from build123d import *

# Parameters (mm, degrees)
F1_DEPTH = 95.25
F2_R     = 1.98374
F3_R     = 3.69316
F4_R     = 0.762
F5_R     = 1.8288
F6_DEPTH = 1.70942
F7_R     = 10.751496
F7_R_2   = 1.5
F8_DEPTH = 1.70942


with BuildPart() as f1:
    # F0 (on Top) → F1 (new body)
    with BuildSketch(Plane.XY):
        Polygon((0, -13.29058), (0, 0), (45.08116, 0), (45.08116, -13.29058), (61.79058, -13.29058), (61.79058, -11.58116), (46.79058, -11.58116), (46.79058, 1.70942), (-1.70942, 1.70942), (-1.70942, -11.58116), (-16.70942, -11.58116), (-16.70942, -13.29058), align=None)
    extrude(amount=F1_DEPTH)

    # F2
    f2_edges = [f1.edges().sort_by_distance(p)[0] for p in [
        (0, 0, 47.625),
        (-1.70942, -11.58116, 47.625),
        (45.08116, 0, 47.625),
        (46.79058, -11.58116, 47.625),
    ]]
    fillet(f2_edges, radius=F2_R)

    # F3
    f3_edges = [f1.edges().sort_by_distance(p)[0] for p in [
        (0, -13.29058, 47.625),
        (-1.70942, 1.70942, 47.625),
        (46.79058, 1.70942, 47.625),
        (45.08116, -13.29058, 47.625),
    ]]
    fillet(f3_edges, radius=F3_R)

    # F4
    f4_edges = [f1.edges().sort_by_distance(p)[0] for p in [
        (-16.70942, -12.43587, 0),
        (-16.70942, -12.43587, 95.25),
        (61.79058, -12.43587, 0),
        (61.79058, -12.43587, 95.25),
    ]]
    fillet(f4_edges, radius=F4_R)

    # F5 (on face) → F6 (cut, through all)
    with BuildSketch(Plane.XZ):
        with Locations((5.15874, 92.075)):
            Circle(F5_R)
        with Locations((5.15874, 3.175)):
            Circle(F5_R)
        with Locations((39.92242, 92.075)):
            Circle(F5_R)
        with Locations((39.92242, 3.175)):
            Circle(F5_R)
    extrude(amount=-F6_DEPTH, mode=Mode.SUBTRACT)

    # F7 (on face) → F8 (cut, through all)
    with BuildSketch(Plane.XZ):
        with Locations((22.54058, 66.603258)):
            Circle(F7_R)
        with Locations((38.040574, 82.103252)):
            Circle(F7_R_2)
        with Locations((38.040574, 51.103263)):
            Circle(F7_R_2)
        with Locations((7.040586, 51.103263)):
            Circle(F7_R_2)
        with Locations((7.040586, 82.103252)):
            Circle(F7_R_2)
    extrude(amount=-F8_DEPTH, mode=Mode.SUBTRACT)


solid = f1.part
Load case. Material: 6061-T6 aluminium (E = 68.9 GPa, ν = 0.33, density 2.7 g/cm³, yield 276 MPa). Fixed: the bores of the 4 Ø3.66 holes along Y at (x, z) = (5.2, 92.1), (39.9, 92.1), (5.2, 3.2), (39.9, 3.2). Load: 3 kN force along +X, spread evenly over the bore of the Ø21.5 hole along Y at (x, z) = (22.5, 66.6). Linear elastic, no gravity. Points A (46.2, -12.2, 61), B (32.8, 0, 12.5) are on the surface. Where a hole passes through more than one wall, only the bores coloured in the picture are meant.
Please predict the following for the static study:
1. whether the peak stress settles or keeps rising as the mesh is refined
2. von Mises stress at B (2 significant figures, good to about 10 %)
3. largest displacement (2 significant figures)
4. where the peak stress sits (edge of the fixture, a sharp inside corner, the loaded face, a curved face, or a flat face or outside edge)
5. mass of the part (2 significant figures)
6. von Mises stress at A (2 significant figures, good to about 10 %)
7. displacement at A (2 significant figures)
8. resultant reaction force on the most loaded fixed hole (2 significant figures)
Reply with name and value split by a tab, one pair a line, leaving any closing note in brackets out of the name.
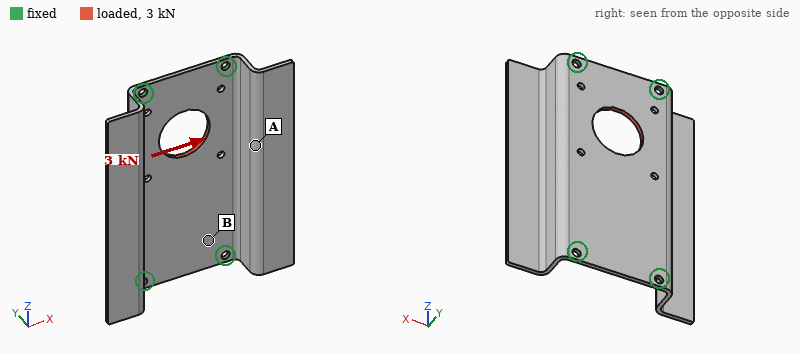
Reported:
whether the peak stress settles or keeps rising as the mesh is refined	keeps rising
von Mises stress at B	32 MPa
largest displacement	56 µm
where the peak stress sits	edge of the fixture
mass of the part	42 g
von Mises stress at A	15 MPa
displacement at A	49 µm
resultant reaction force on the most loaded fixed hole	1.1 kN
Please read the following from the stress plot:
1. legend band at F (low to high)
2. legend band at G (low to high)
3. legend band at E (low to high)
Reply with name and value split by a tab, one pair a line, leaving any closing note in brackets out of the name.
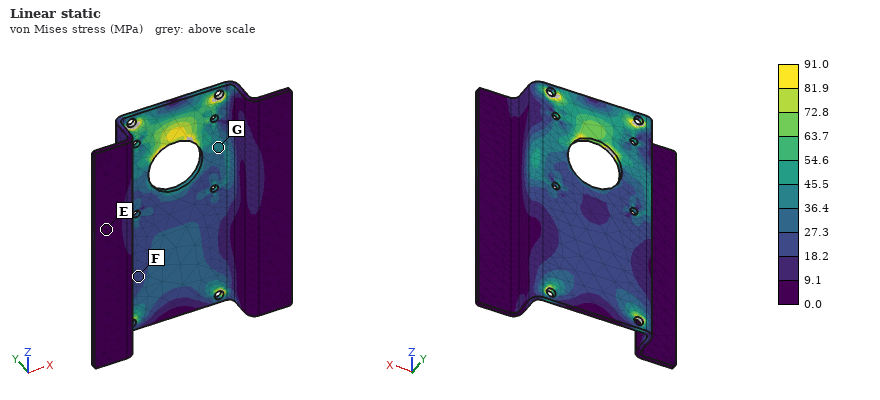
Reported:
legend band at F	18.2 to 27.3 MPa
legend band at G	36.4 to 45.5 MPa
legend band at E	0.0 to 9.1 MPa
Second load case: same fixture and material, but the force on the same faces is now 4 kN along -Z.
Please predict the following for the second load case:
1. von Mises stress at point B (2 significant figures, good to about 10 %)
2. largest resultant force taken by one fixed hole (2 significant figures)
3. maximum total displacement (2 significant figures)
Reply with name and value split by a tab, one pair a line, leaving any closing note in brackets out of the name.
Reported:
von Mises stress at point B	19 MPa
largest resultant force taken by one fixed hole	1.3 kN
maximum total displacement	21 µm
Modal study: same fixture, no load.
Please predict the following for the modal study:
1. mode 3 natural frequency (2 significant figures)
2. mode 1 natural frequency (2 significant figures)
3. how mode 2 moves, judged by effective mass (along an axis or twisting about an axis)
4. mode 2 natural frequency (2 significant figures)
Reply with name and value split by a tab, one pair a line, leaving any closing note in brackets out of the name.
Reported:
mode 3 natural frequency	2100 Hz
mode 1 natural frequency	1300 Hz
how mode 2 moves, judged by effective mass	along X
mode 2 natural frequency	1500 Hz
